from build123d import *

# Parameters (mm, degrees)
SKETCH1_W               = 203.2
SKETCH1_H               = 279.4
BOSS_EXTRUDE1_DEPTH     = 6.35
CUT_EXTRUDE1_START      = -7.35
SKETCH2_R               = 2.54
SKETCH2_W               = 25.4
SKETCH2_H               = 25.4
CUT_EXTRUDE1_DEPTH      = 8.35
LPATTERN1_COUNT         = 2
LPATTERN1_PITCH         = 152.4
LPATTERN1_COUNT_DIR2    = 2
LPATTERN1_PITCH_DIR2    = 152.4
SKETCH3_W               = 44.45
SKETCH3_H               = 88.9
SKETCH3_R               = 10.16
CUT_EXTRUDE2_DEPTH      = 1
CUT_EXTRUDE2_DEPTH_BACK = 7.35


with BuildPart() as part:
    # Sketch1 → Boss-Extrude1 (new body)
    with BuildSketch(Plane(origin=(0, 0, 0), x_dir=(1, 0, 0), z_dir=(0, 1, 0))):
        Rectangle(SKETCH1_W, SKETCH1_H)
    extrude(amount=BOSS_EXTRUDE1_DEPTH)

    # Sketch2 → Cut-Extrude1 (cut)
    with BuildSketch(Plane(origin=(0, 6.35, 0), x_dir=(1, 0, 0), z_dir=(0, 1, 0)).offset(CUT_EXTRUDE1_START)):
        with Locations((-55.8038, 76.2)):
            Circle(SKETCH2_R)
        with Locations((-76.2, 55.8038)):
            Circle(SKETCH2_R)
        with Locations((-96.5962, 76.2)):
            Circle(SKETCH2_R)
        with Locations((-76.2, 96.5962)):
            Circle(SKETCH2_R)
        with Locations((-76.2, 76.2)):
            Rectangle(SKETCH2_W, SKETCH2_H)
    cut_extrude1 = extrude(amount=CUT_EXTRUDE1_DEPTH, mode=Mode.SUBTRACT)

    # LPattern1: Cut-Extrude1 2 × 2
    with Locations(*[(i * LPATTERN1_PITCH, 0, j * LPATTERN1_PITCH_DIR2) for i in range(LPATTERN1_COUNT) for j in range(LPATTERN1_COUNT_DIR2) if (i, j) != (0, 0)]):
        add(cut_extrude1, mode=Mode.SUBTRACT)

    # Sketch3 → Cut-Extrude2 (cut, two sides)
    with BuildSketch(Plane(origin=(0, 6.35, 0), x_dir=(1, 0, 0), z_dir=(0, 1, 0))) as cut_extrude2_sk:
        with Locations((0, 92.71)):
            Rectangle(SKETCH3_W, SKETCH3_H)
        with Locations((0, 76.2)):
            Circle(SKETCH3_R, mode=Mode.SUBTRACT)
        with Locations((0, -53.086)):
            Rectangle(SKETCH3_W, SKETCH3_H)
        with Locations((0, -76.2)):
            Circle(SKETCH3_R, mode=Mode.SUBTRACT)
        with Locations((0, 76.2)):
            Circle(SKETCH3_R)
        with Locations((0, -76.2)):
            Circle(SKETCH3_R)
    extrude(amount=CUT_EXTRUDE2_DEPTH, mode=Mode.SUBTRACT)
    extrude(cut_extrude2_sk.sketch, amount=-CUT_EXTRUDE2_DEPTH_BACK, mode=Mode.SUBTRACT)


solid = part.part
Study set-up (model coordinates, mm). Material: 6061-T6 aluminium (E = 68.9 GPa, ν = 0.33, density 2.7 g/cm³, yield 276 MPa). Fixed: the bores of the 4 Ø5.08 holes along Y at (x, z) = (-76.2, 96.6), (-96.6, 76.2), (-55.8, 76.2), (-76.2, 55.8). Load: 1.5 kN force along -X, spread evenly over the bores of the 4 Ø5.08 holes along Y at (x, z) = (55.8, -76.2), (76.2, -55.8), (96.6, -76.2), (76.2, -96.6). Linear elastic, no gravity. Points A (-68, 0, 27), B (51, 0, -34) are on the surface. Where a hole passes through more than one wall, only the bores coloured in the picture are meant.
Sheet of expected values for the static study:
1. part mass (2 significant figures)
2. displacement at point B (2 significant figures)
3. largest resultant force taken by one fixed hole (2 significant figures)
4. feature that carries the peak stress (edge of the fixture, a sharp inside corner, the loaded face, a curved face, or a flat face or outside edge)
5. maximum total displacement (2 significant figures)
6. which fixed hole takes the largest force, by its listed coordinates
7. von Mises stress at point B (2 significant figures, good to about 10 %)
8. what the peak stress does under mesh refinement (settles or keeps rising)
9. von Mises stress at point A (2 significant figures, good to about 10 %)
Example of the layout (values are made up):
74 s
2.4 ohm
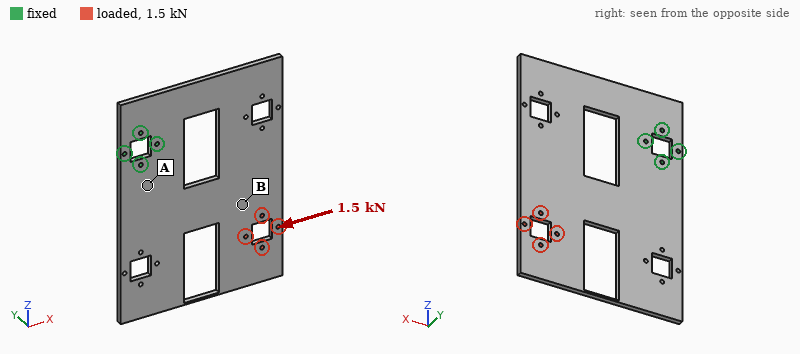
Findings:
790 g
0.097 mm
3.5 kN
edge of the fixture
0.18 mm
(-55.8, 76.2)
4.4 MPa
keeps rising
10 MPa
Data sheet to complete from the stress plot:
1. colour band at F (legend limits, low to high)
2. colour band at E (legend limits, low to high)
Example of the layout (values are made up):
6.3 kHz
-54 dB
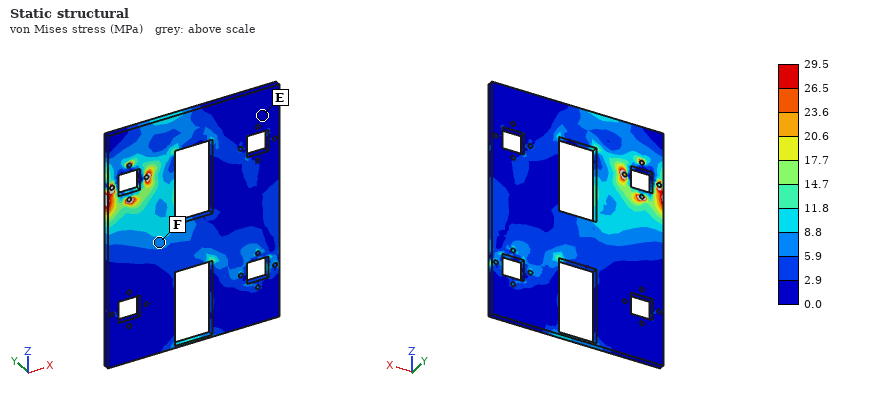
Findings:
5.9 to 8.8 MPa
0.0 to 2.9 MPa
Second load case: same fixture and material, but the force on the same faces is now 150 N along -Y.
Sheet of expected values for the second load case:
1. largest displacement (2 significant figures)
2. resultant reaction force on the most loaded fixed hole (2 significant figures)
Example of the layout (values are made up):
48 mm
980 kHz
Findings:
3.5 mm
320 N
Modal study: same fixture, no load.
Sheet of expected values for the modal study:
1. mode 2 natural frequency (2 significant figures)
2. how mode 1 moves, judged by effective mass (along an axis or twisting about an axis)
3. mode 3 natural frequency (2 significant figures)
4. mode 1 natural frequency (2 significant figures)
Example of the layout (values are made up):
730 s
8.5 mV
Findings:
160 Hz
along Y
290 Hz
86 Hz
